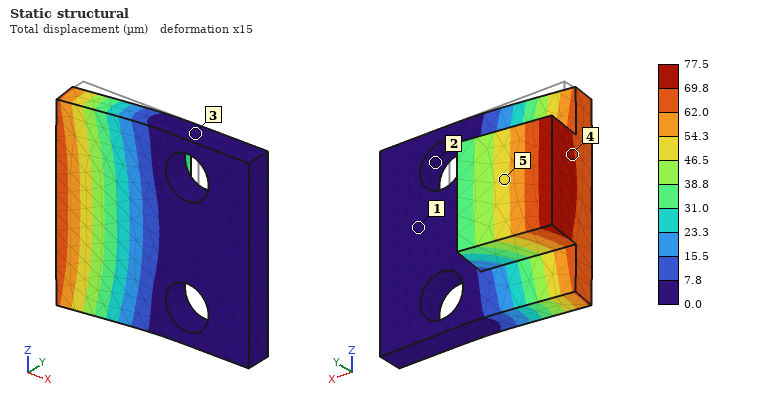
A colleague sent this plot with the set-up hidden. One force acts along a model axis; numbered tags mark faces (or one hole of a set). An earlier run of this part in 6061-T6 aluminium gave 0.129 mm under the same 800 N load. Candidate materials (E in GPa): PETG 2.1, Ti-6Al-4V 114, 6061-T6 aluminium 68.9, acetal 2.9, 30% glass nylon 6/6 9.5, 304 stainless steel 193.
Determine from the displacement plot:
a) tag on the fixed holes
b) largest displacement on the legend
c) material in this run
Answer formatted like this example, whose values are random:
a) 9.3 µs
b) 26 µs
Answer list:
a) 2
b) 77.5 µm
c) Ti-6Al-4V
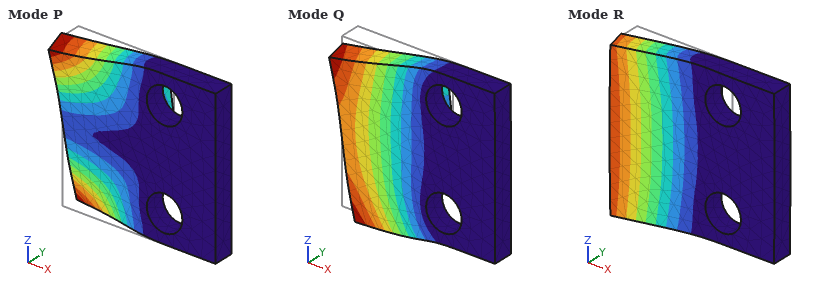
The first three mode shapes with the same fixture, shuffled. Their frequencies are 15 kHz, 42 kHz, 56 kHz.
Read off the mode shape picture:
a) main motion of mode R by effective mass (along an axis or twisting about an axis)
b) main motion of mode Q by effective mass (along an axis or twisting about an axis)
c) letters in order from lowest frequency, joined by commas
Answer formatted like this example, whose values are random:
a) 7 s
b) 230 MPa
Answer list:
a) along Y
b) along Z
c) R, P, Q
